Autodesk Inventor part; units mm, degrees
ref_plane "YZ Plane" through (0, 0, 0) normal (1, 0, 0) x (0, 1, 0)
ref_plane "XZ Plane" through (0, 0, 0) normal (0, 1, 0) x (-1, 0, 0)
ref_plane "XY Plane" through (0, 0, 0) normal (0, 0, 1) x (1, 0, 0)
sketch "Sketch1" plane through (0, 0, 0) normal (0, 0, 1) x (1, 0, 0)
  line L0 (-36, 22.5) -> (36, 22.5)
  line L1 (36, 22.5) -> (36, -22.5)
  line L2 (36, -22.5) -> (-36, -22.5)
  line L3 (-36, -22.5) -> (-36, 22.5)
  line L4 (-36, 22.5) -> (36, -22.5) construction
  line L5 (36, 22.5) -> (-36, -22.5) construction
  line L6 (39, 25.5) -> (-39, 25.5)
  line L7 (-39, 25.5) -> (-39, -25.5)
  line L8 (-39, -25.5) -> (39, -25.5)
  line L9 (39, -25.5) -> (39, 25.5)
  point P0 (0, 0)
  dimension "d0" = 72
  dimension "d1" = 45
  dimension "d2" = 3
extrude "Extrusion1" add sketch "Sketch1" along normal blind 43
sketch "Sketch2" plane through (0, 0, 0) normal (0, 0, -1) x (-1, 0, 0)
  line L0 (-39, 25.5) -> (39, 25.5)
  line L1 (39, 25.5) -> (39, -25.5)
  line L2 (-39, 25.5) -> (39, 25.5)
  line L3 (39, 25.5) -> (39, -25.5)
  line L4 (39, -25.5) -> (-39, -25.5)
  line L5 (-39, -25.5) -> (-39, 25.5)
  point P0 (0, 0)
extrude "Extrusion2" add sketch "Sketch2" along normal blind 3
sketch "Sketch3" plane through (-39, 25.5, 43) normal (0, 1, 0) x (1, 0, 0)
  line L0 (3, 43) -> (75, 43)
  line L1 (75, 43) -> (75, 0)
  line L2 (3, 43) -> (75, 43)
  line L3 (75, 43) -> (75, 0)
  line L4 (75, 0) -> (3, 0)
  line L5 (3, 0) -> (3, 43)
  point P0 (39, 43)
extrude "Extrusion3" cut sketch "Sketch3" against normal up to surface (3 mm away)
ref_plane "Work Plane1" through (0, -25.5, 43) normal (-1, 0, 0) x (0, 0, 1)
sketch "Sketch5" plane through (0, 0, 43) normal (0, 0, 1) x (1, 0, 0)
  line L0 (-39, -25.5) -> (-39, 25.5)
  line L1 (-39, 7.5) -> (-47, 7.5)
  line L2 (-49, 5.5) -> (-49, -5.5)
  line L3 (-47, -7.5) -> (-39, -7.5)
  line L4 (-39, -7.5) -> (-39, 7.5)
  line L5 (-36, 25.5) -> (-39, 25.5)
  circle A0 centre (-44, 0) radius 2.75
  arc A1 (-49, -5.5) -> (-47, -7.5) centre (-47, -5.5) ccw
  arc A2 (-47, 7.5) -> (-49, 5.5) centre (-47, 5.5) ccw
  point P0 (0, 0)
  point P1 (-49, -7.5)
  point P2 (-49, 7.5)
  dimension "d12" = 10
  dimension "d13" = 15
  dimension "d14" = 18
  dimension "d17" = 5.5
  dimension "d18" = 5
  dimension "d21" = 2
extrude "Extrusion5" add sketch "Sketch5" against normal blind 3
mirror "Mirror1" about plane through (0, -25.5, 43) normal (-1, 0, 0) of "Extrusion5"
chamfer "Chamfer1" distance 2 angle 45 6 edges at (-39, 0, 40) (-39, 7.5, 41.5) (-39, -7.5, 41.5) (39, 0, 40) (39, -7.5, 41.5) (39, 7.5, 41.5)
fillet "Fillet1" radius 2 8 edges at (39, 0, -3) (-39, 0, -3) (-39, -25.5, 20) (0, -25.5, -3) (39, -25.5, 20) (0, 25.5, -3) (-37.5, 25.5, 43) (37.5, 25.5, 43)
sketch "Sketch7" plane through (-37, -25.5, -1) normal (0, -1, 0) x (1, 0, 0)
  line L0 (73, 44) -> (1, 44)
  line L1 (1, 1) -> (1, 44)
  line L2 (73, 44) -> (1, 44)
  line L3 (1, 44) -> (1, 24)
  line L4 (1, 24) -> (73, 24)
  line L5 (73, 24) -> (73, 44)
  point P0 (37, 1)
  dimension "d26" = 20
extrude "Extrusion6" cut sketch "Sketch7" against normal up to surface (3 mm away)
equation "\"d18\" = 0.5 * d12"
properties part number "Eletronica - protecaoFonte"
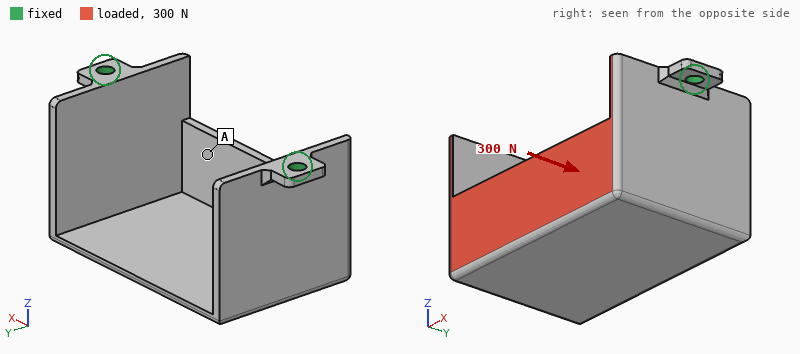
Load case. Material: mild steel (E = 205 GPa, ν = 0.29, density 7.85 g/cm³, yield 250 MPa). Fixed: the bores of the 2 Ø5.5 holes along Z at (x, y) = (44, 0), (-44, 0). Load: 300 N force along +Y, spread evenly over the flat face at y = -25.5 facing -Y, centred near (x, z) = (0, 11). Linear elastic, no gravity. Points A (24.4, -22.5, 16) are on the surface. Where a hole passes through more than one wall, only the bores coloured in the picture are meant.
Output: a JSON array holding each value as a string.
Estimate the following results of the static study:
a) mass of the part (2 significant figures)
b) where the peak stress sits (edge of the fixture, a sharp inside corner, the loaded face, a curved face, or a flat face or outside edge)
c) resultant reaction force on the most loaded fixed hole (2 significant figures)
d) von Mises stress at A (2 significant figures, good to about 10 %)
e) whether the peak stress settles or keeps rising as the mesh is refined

["240 g", "edge of the fixture", "150 N", "11 MPa", "keeps rising"]
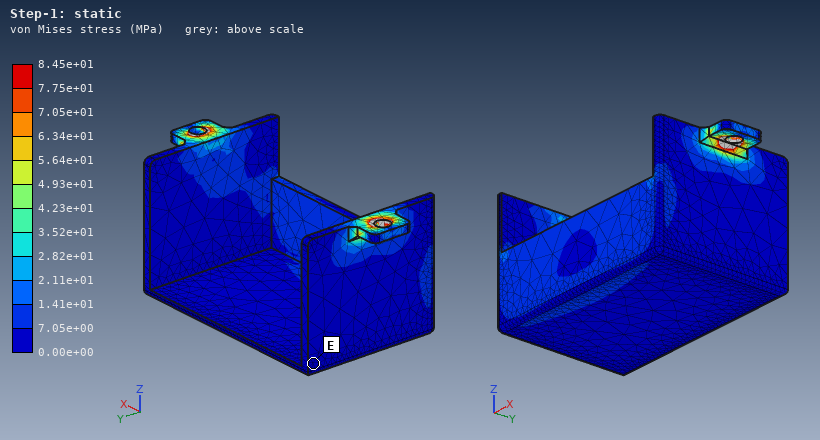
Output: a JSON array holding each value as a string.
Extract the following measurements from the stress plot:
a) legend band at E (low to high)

["0.00e+00 to 7.05e+00 MPa"]
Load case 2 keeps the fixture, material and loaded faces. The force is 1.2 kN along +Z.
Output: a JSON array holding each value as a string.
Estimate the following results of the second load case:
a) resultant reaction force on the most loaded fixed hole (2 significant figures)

["610 N"]
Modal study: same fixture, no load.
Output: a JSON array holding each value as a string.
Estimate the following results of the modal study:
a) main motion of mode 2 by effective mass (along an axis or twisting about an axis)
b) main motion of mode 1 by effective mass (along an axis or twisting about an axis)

["along X", "along Y"]
